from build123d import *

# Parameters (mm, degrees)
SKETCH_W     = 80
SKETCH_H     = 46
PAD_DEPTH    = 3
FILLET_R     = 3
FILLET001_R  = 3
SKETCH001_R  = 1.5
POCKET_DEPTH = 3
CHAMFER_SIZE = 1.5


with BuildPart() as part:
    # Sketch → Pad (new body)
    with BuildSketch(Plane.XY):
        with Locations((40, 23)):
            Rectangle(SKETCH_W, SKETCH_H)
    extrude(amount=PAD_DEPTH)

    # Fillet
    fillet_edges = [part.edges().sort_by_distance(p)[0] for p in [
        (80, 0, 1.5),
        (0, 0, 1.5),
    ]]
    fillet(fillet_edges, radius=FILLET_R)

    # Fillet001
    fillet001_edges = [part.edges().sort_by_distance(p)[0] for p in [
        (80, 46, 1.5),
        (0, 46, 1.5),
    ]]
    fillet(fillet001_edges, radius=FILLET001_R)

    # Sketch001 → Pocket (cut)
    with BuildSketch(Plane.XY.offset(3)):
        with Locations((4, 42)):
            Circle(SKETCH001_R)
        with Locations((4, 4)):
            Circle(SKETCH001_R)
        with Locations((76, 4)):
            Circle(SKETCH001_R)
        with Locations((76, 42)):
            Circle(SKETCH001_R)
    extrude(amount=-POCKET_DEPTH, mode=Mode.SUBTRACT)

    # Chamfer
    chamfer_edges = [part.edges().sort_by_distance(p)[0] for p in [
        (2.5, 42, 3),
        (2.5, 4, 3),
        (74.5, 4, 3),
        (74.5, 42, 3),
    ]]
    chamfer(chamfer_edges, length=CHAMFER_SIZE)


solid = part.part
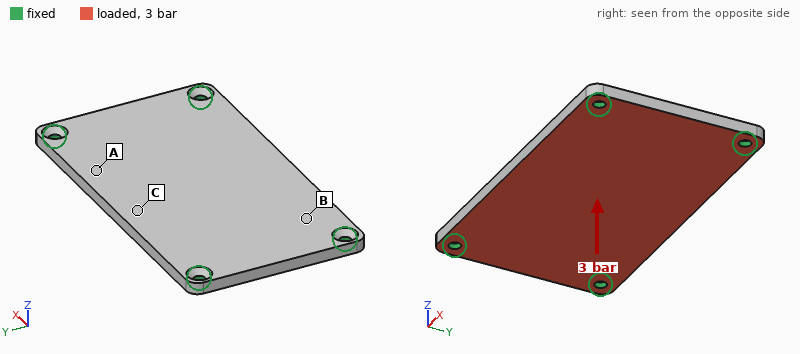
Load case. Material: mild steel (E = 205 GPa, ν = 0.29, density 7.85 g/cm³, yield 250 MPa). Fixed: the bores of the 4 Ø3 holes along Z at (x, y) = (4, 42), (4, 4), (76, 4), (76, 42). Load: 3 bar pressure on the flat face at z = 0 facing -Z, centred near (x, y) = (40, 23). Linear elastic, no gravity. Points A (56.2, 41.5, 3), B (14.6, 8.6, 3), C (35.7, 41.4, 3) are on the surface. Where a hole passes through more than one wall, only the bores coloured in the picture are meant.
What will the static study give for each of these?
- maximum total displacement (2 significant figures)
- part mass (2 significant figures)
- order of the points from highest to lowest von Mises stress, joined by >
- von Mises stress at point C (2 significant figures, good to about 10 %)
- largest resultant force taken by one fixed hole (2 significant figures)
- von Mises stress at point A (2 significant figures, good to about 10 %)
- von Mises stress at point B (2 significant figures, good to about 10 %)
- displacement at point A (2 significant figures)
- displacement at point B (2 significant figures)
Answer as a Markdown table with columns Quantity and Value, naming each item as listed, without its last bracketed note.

| Quantity | Value |
|---|---|
| maximum total displacement | 80 µm |
| part mass | 85 g |
| order of the points from highest to lowest von Mises stress, joined by > | C > A > B |
| von Mises stress at point C | 63 MPa |
| largest resultant force taken by one fixed hole | 440 N |
| von Mises stress at point A | 42 MPa |
| von Mises stress at point B | 21 MPa |
| displacement at point A | 55 µm |
| displacement at point B | 30 µm |
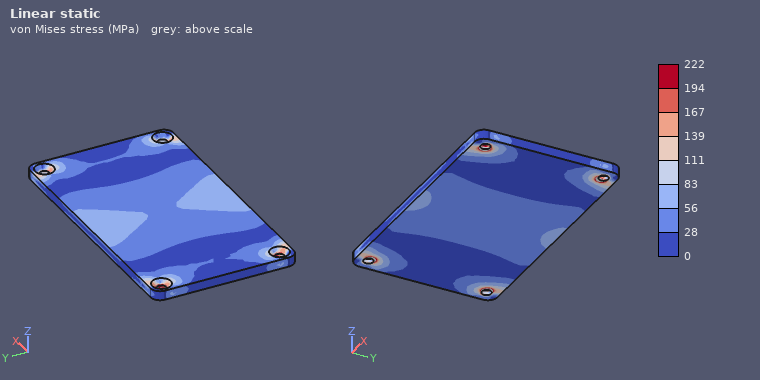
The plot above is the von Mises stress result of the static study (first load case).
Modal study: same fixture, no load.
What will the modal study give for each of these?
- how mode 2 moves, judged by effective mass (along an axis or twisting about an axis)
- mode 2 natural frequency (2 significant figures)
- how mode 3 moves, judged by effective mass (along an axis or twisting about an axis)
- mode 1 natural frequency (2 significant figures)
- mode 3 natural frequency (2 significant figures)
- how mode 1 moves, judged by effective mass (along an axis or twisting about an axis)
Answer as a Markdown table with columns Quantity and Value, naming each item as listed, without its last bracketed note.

| Quantity | Value |
|---|---|
| how mode 2 moves, judged by effective mass | twisting about X |
| mode 2 natural frequency | 4000 Hz |
| how mode 3 moves, judged by effective mass | twisting about Y |
| mode 1 natural frequency | 2300 Hz |
| mode 3 natural frequency | 6200 Hz |
| how mode 1 moves, judged by effective mass | along Z |
